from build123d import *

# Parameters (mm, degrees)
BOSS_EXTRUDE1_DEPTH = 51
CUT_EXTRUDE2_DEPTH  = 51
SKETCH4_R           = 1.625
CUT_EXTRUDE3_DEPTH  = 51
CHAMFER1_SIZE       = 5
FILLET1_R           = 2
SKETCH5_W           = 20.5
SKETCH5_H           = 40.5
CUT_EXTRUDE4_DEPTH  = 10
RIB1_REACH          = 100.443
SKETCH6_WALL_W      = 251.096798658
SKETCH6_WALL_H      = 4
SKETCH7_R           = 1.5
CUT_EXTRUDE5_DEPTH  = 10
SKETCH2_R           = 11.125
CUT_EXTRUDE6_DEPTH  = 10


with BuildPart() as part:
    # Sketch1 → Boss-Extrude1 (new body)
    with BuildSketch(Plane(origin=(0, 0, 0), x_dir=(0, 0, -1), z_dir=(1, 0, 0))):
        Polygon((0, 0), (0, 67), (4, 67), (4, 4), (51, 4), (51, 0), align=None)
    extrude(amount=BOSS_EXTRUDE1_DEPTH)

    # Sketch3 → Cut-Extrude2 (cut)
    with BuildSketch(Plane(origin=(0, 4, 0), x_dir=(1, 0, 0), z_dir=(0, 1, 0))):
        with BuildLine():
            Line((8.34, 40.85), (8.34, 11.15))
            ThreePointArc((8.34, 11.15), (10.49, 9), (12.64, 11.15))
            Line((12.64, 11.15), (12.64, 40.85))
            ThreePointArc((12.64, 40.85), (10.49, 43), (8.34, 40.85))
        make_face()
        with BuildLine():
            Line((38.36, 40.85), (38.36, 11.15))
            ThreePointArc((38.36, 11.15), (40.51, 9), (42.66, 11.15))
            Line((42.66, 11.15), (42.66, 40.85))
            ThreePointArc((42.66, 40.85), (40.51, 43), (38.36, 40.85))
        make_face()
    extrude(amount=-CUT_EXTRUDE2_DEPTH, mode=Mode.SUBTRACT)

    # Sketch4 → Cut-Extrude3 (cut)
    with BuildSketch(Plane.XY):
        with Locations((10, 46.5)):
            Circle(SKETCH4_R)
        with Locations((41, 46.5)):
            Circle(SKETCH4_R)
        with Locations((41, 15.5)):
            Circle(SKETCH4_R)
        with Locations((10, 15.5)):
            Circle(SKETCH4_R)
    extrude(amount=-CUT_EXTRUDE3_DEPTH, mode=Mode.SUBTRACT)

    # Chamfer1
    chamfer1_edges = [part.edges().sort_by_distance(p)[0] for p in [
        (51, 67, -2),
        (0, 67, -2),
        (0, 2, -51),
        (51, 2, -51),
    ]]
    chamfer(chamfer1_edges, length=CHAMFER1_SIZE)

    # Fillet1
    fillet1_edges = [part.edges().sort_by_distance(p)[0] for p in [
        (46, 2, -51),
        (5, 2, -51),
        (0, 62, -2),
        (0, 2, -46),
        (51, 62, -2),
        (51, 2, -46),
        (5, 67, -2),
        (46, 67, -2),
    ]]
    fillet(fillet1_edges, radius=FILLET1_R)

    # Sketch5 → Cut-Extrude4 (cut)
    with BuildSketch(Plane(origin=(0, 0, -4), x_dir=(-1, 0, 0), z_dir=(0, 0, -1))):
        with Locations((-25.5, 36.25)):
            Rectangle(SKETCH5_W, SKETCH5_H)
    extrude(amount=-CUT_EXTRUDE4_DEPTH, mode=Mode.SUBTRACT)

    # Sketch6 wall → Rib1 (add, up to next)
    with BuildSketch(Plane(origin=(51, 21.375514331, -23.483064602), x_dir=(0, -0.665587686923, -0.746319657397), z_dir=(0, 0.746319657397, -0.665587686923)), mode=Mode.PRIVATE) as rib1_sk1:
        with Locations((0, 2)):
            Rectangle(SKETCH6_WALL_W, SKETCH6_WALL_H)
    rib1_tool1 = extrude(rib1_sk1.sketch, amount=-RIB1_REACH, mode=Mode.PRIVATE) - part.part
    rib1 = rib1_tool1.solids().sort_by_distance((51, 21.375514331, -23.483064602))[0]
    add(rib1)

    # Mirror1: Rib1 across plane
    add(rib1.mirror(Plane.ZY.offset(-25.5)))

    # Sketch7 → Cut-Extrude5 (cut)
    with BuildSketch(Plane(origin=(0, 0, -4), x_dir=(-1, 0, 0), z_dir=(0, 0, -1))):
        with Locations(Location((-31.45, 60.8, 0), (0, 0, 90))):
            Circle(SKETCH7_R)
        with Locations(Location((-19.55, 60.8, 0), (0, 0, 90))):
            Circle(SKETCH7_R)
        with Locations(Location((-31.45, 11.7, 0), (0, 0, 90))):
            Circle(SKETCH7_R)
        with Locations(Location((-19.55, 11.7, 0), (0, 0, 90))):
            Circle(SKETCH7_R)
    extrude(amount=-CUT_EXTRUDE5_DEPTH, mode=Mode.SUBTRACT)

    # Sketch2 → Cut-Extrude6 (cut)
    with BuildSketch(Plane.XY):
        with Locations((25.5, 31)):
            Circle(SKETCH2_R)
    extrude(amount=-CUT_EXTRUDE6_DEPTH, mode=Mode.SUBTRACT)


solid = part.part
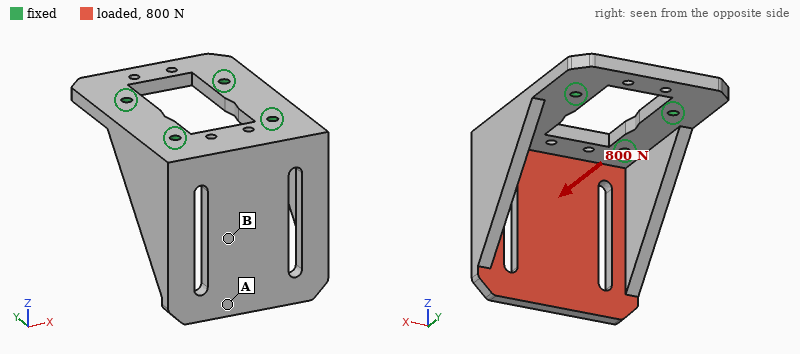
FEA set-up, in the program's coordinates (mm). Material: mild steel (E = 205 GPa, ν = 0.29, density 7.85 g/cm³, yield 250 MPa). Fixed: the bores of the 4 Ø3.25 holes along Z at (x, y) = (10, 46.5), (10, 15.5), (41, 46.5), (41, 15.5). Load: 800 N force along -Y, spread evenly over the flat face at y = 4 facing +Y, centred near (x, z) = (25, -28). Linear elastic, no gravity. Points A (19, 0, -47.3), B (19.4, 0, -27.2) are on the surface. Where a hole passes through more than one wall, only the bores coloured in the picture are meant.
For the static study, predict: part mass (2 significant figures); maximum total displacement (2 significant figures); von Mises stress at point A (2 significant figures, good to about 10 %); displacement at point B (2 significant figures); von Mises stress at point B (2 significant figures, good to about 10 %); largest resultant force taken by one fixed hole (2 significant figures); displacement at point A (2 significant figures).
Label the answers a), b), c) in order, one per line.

a) 190 g
b) 55 µm
c) 34 MPa
d) 32 µm
e) 14 MPa
f) 440 N
g) 49 µm
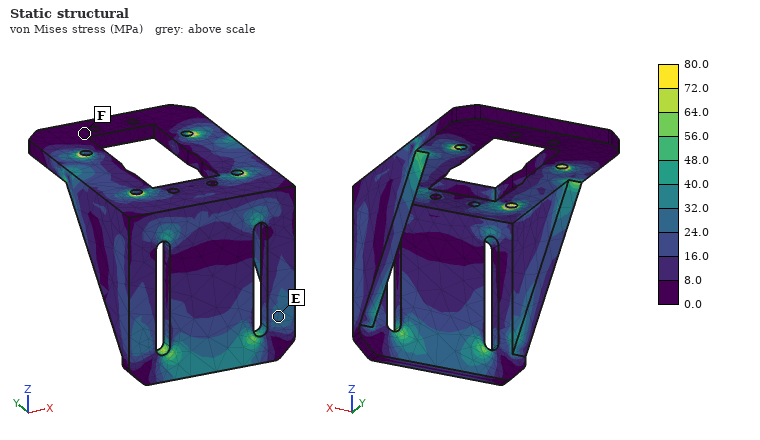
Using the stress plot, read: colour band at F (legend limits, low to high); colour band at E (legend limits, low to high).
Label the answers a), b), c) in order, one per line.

a) 0.0 to 8.0 MPa
b) 24.0 to 32.0 MPa
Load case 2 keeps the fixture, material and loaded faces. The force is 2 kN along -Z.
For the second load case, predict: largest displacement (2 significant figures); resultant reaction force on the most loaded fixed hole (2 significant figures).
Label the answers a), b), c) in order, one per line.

a) 30 µm
b) 1.3 kN
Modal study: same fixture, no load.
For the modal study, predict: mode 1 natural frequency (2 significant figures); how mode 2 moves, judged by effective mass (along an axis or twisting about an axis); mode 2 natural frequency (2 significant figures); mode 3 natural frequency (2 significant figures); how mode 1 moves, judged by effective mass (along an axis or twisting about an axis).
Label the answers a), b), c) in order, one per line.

a) 2900 Hz
b) along X
c) 3200 Hz
d) 6000 Hz
e) along Y
